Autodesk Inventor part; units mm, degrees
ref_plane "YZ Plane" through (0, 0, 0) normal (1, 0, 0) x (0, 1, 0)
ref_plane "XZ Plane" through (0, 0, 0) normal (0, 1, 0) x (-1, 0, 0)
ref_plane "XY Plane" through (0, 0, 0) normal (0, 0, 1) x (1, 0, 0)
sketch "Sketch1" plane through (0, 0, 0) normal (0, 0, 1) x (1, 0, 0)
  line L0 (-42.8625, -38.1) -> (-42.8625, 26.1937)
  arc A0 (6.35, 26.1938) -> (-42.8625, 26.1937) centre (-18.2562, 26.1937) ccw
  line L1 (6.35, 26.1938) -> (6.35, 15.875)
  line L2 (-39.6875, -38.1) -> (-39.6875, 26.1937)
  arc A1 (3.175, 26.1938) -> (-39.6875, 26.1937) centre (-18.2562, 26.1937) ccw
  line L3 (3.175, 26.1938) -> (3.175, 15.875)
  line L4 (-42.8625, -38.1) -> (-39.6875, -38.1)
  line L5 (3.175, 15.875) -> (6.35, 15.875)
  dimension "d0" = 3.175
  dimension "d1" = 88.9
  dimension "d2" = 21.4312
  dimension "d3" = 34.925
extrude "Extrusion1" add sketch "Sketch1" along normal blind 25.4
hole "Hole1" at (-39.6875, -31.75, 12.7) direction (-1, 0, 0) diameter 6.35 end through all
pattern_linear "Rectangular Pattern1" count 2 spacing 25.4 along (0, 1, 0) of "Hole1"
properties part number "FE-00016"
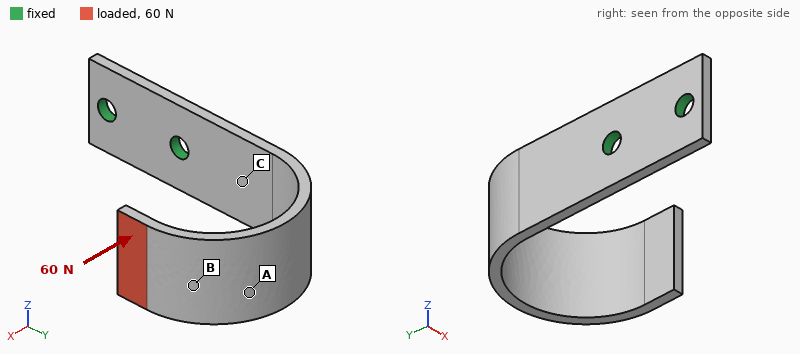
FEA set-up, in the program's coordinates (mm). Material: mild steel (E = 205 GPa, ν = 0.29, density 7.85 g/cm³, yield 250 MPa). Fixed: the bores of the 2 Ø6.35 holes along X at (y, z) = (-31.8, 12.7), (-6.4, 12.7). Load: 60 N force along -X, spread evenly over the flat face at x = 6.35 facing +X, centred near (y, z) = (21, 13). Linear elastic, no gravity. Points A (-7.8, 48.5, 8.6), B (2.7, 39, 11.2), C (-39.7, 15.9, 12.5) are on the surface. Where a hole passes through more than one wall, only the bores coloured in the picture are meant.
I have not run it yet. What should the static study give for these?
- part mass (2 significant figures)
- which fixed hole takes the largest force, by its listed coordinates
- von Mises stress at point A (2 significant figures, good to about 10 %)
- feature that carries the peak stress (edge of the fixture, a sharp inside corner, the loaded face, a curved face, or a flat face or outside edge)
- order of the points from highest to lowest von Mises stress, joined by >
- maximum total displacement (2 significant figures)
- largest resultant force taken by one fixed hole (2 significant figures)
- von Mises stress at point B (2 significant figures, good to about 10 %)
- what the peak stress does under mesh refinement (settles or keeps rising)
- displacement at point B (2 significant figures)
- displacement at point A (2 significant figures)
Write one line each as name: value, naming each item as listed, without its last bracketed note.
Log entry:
part mass: 91 g
which fixed hole takes the largest force, by its listed coordinates: (-6.4, 12.7)
von Mises stress at point A: 31 MPa
feature that carries the peak stress: edge of the fixture
order of the points from highest to lowest von Mises stress, joined by >: A > B > C
maximum total displacement: 0.20 mm
largest resultant force taken by one fixed hole: 67 N
von Mises stress at point B: 20 MPa
what the peak stress does under mesh refinement: keeps rising
displacement at point B: 0.10 mm
displacement at point A: 0.056 mm
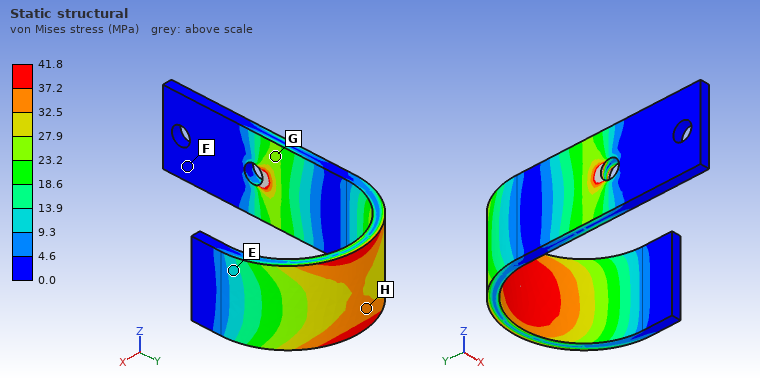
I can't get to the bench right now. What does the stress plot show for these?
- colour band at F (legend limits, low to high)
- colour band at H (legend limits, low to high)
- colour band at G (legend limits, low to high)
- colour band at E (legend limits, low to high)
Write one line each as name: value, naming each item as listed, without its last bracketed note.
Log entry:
colour band at F: 0.0 to 4.6 MPa
colour band at H: 32.5 to 37.2 MPa
colour band at G: 23.2 to 27.9 MPa
colour band at E: 9.3 to 13.9 MPa
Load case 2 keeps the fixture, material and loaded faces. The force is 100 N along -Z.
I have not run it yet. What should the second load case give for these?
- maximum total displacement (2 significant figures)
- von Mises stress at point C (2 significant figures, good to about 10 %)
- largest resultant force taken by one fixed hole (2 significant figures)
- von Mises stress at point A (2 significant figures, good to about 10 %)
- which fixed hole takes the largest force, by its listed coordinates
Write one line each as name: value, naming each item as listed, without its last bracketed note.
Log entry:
maximum total displacement: 0.75 mm
von Mises stress at point C: 110 MPa
largest resultant force taken by one fixed hole: 160 N
von Mises stress at point A: 36 MPa
which fixed hole takes the largest force, by its listed coordinates: (-6.4, 12.7)
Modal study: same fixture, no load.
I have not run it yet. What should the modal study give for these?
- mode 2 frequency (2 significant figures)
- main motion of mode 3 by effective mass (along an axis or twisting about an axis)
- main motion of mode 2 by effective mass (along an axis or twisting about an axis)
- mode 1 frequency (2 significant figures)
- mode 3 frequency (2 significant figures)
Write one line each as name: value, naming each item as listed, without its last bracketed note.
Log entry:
mode 2 frequency: 440 Hz
main motion of mode 3 by effective mass: along X
main motion of mode 2 by effective mass: along Z
mode 1 frequency: 300 Hz
mode 3 frequency: 700 Hz
